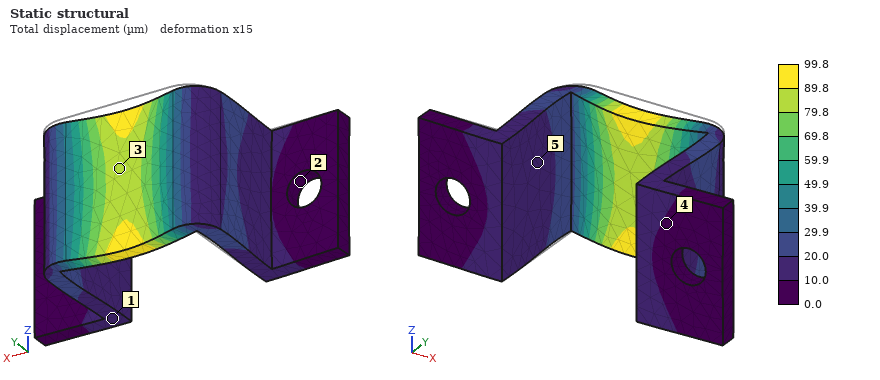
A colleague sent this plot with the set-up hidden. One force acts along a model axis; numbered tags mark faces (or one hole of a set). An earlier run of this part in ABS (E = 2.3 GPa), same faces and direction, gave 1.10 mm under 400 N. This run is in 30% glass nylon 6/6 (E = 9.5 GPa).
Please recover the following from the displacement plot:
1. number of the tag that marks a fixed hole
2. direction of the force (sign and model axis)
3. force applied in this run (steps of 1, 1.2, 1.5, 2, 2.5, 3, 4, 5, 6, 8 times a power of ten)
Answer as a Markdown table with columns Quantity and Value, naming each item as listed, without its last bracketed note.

| Quantity | Value |
|---|---|
| number of the tag that marks a fixed hole | 2 |
| direction of the force | -Y |
| force applied in this run | 150 N |
